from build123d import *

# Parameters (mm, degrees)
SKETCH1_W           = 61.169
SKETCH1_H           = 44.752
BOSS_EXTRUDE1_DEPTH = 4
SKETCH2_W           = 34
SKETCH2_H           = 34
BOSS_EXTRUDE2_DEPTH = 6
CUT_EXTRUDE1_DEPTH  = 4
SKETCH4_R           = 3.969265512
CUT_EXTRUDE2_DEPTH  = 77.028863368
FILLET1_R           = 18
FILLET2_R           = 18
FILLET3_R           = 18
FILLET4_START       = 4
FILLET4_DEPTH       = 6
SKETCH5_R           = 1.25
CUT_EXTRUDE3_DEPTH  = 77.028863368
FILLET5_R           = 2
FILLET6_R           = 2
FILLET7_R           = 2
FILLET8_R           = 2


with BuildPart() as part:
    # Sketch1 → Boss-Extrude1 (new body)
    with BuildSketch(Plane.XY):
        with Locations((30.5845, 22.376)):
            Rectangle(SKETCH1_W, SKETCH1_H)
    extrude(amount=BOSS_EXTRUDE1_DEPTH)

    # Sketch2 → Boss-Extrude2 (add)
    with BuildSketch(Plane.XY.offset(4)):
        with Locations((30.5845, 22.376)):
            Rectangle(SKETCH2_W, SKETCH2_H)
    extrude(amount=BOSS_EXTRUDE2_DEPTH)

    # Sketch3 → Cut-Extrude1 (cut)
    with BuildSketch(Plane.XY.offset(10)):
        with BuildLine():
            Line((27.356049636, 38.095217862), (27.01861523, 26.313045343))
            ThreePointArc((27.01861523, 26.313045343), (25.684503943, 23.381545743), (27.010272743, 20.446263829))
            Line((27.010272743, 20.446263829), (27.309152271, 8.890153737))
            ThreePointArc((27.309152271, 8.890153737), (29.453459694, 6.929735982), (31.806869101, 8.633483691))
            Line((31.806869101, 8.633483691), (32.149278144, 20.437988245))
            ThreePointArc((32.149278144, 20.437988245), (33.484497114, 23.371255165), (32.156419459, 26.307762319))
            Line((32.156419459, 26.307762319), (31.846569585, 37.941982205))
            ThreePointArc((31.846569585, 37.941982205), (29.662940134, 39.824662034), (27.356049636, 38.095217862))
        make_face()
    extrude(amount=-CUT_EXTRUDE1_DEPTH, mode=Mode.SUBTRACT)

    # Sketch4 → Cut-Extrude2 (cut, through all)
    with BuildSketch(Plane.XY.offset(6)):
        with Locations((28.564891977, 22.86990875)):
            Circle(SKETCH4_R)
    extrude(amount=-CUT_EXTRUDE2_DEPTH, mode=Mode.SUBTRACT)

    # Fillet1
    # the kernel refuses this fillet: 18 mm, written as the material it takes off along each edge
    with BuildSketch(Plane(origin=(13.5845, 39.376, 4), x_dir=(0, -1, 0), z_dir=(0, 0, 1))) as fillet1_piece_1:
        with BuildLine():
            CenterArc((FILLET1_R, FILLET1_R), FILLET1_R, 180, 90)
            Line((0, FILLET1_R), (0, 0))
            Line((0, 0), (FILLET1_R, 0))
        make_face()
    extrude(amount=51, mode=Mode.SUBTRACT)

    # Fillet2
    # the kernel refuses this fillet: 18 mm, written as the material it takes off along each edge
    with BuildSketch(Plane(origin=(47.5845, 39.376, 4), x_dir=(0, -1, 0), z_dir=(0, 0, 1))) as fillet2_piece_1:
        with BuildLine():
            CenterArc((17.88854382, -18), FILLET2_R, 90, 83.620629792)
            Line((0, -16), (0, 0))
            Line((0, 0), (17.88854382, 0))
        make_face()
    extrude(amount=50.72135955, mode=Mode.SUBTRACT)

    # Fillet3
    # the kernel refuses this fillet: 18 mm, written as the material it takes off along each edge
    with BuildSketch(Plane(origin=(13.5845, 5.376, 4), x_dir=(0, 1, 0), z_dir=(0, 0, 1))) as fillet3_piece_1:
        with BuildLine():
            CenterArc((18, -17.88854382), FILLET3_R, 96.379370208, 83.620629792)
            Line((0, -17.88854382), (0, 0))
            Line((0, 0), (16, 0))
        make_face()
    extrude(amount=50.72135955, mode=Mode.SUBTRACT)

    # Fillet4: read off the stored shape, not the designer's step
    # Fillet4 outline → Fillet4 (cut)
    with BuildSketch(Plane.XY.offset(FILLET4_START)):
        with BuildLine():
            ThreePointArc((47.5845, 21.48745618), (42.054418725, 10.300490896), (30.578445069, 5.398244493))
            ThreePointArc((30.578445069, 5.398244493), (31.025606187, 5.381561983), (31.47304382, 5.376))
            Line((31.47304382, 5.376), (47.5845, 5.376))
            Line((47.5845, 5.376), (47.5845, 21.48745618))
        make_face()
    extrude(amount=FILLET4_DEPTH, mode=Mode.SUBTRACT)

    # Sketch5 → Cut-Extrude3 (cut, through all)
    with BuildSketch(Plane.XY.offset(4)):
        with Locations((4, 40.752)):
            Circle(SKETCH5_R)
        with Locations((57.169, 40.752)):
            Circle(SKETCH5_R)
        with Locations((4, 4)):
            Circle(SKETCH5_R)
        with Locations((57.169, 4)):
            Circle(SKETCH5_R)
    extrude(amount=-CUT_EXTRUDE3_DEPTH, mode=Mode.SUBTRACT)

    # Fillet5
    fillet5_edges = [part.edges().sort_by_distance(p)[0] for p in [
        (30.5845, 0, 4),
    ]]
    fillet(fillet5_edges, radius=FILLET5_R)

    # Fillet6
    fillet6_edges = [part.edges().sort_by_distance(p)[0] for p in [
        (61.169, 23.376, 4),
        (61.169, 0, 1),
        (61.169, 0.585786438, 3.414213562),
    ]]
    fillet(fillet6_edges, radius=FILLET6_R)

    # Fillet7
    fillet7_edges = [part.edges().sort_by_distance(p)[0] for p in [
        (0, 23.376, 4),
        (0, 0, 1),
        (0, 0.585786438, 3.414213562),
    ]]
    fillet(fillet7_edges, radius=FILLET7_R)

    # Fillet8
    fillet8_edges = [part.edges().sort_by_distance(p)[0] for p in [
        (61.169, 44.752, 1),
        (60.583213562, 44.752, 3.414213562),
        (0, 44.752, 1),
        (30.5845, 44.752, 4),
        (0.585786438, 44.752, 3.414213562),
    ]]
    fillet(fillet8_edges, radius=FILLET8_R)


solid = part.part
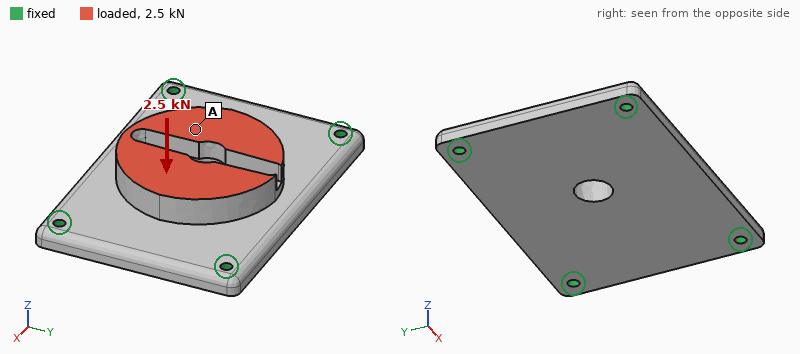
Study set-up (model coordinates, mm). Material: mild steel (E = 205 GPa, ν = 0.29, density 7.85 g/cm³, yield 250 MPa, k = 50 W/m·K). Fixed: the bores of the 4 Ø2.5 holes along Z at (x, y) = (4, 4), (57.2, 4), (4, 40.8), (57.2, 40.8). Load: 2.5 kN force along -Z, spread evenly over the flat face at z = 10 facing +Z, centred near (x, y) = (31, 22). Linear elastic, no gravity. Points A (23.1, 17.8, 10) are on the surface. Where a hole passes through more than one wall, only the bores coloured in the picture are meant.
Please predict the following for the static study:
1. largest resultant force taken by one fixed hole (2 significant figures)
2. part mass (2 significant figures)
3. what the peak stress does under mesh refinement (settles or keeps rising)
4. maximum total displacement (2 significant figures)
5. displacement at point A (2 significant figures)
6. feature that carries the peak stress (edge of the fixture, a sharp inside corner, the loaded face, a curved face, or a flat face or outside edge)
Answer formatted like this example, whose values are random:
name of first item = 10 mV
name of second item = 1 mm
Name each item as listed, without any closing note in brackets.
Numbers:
largest resultant force taken by one fixed hole = 730 N
part mass = 120 g
what the peak stress does under mesh refinement = keeps rising
maximum total displacement = 29 µm
displacement at point A = 26 µm
feature that carries the peak stress = edge of the fixture
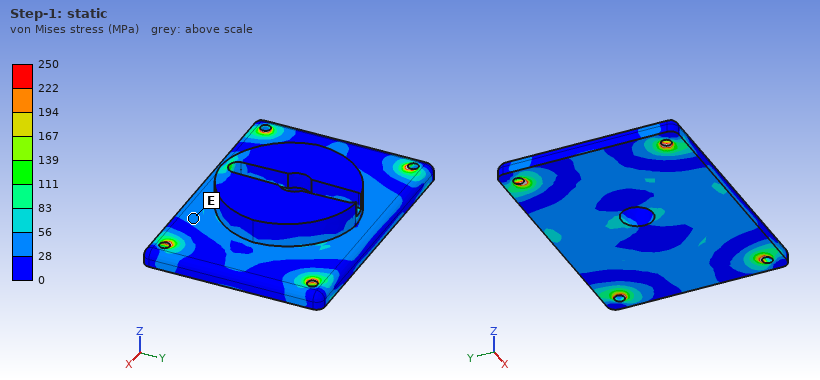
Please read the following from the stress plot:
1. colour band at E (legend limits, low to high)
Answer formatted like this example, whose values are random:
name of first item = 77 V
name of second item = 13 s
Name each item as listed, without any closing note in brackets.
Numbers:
colour band at E = 28 to 56 MPa
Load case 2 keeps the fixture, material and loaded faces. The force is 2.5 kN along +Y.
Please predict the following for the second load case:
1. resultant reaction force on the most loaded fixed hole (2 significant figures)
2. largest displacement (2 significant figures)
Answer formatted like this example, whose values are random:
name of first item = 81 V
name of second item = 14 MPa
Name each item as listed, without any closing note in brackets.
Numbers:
resultant reaction force on the most loaded fixed hole = 810 N
largest displacement = 15 µm
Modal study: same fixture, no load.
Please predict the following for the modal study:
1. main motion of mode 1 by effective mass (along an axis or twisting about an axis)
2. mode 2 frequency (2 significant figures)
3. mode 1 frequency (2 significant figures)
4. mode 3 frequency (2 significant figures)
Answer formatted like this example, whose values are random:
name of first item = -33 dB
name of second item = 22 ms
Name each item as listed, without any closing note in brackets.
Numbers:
main motion of mode 1 by effective mass = along Z
mode 2 frequency = 8500 Hz
mode 1 frequency = 5400 Hz
mode 3 frequency = 12 kHz
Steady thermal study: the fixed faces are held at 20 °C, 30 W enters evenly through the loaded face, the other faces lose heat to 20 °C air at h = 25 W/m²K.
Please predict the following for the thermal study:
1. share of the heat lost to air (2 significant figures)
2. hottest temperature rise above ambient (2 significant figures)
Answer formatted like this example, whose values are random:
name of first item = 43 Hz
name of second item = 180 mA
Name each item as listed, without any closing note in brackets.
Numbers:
share of the heat lost to air = 14 %
hottest temperature rise above ambient = 44 K
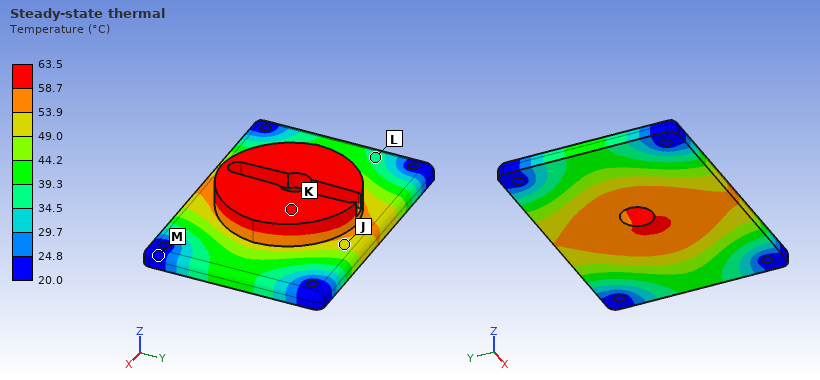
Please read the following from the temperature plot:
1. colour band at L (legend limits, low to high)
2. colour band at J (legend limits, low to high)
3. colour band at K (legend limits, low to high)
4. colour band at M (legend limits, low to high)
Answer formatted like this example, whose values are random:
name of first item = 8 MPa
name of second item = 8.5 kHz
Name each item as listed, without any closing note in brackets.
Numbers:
colour band at L = 34.5 to 39.3 °C
colour band at J = 49.0 to 53.9 °C
colour band at K = 58.7 to 63.5 °C
colour band at M = 20.0 to 24.8 °C
